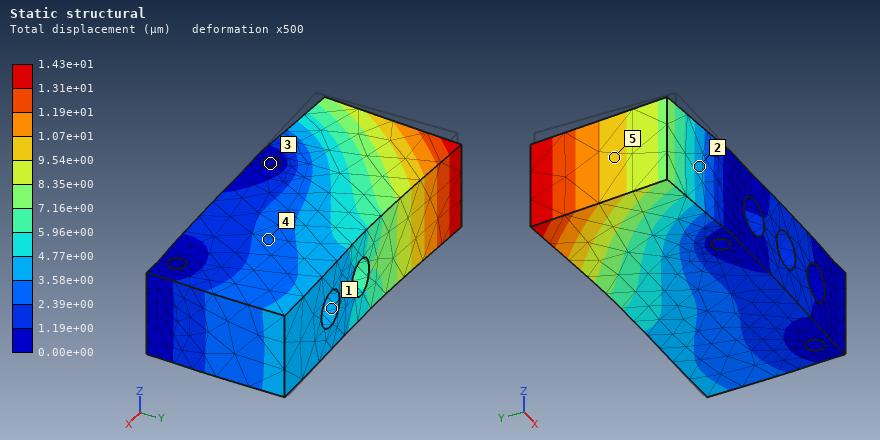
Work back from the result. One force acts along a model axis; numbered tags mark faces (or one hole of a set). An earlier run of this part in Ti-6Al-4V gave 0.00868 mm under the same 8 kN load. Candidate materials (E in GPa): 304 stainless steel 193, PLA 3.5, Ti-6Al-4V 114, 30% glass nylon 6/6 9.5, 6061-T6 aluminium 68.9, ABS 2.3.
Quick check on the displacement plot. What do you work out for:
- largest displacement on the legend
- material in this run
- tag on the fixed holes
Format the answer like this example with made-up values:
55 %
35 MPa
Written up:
1.43e+01 µm
6061-T6 aluminium
3
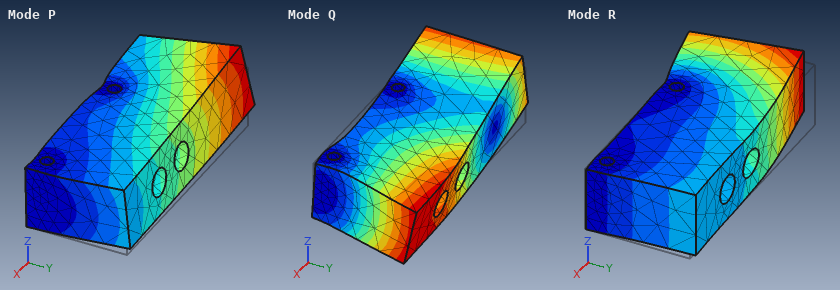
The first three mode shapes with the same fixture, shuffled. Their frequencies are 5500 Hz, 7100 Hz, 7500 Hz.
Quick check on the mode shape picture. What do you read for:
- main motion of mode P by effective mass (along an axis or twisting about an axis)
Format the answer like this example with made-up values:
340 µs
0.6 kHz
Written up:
along Z
